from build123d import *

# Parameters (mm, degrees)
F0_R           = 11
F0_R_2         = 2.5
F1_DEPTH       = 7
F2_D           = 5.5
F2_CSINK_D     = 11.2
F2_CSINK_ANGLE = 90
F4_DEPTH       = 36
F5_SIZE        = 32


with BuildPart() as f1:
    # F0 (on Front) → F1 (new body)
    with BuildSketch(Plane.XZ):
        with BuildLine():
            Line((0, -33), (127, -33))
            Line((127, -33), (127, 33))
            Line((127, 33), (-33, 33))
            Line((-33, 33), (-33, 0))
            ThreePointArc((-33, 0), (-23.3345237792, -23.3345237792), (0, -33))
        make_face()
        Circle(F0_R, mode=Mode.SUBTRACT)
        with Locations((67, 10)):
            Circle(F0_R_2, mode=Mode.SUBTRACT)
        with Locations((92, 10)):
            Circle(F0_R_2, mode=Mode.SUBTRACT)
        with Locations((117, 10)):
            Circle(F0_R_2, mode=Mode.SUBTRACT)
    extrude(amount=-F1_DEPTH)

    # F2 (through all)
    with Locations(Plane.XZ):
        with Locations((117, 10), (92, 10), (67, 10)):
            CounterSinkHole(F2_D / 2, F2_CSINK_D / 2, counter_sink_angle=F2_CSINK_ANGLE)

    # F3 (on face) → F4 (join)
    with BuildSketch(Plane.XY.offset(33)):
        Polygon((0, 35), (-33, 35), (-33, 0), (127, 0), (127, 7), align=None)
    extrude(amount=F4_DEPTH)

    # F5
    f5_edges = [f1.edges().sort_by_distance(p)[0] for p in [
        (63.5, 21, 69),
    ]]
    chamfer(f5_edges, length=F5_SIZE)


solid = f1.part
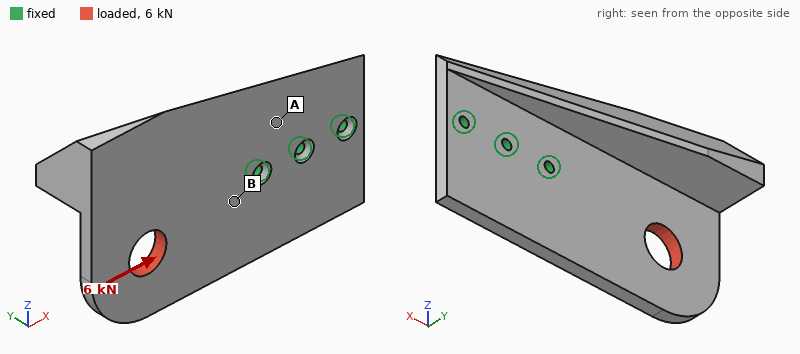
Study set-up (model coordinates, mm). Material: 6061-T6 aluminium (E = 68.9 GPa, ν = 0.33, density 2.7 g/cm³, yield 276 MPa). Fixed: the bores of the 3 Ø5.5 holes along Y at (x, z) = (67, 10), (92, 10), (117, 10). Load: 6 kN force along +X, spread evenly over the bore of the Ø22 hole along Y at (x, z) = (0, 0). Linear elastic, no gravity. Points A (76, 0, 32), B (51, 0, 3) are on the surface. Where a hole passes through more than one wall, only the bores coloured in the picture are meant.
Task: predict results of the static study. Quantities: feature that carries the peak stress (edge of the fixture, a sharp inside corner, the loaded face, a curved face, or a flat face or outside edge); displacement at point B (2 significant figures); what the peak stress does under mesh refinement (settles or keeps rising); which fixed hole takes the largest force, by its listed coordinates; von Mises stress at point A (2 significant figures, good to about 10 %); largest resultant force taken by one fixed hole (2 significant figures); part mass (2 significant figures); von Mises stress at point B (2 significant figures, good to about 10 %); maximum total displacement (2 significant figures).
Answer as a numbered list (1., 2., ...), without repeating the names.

1. edge of the fixture
2. 11 µm
3. keeps rising
4. (67, 10)
5. 4.7 MPa
6. 3.6 kN
7. 370 g
8. 16 MPa
9. 48 µm
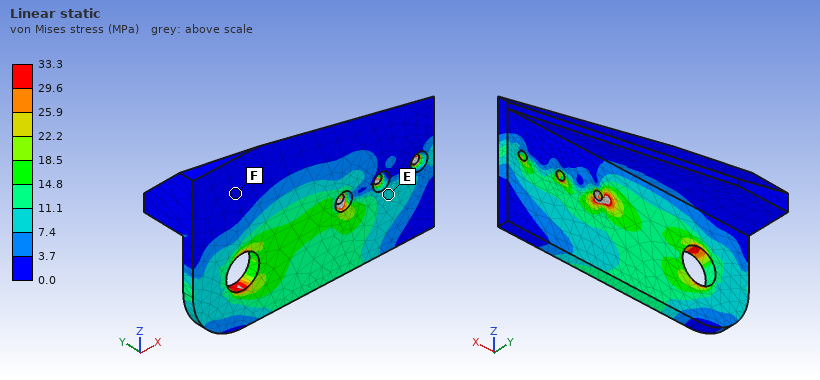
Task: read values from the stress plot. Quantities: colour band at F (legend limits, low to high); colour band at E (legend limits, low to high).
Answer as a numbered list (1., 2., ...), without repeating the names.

1. 0.0 to 3.7 MPa
2. 7.4 to 11.1 MPa
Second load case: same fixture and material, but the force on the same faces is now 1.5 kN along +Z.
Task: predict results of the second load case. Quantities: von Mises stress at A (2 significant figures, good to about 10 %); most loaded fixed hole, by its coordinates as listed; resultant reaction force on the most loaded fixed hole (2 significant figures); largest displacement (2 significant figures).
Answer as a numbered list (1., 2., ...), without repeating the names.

1. 7.7 MPa
2. (67, 10)
3. 3.4 kN
4. 59 µm
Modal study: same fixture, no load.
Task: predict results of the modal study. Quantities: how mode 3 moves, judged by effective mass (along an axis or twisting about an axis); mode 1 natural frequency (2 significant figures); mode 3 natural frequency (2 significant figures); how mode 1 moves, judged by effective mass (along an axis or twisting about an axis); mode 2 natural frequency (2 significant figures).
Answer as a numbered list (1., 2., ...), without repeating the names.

1. along Z
2. 460 Hz
3. 1900 Hz
4. along Y
5. 960 Hz
